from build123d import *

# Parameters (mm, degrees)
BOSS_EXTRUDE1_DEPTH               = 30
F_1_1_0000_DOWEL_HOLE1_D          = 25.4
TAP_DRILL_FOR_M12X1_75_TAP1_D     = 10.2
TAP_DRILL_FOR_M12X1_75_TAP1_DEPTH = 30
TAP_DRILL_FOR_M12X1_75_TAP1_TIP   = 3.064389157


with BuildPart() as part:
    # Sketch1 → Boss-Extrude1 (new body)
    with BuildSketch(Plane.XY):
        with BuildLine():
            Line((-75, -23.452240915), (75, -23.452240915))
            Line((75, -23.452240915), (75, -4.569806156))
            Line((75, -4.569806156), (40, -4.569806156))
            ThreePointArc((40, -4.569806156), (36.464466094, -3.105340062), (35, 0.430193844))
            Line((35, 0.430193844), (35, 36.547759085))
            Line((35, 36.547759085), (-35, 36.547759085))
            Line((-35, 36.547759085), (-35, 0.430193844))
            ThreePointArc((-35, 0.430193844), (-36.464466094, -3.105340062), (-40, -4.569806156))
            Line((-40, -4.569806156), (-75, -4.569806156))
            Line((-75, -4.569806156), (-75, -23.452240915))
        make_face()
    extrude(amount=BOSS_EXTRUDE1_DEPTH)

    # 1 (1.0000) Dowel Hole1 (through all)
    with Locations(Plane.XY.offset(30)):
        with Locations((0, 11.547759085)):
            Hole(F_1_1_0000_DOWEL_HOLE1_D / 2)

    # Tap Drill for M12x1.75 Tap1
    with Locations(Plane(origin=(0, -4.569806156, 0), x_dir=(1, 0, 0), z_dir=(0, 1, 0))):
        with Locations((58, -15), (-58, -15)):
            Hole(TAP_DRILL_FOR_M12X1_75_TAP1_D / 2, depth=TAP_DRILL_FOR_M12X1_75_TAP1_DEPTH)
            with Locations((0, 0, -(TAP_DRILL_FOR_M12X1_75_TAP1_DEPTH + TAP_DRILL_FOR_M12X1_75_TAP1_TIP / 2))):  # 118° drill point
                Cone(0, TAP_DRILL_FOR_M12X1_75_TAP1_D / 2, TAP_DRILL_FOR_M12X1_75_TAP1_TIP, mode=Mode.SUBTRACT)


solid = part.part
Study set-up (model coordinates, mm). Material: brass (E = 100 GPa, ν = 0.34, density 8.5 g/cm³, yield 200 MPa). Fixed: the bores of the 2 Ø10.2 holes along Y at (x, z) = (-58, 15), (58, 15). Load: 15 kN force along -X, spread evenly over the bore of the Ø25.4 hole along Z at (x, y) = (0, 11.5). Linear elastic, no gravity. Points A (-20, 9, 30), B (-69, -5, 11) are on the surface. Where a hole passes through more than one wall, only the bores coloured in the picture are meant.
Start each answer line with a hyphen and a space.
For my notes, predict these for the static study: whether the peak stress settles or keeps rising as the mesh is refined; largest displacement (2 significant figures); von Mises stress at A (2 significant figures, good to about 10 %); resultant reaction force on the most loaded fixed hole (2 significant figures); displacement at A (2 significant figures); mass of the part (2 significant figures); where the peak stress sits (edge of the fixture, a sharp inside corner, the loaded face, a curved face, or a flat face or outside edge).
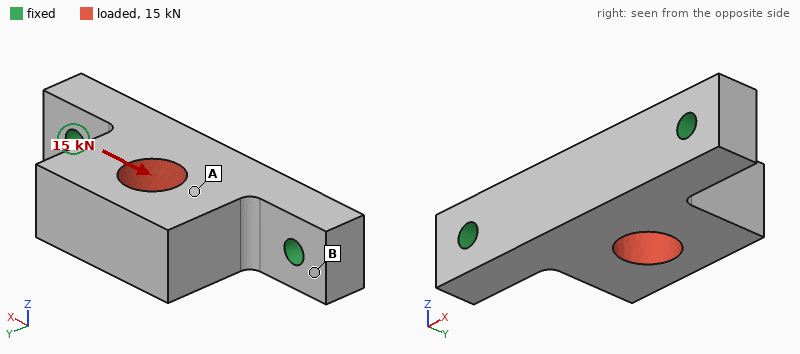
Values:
- keeps rising
- 24 µm
- 18 MPa
- 8.5 kN
- 12 µm
- 1.3 kg
- edge of the fixture
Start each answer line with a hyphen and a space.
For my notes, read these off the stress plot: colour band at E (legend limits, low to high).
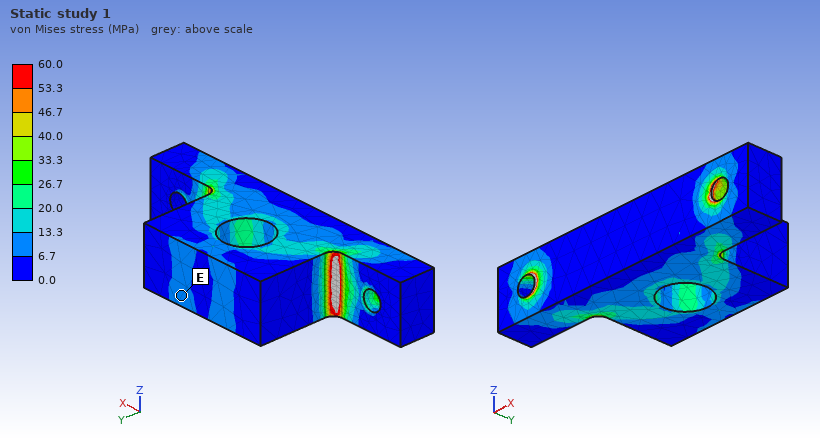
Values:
- 6.7 to 13.3 MPa
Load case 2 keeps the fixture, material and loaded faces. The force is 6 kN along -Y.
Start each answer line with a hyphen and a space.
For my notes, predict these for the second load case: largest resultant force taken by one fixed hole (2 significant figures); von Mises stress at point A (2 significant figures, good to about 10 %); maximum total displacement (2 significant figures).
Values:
- 3.3 kN
- 6.0 MPa
- 12 µm
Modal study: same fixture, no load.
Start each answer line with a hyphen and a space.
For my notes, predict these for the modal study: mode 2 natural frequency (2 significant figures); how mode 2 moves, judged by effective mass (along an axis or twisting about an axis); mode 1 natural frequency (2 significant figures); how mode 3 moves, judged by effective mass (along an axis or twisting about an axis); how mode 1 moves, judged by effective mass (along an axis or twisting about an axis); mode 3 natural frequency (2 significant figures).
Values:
- 4000 Hz
- along Y
- 1800 Hz
- along Z
- along Z
- 5000 Hz
